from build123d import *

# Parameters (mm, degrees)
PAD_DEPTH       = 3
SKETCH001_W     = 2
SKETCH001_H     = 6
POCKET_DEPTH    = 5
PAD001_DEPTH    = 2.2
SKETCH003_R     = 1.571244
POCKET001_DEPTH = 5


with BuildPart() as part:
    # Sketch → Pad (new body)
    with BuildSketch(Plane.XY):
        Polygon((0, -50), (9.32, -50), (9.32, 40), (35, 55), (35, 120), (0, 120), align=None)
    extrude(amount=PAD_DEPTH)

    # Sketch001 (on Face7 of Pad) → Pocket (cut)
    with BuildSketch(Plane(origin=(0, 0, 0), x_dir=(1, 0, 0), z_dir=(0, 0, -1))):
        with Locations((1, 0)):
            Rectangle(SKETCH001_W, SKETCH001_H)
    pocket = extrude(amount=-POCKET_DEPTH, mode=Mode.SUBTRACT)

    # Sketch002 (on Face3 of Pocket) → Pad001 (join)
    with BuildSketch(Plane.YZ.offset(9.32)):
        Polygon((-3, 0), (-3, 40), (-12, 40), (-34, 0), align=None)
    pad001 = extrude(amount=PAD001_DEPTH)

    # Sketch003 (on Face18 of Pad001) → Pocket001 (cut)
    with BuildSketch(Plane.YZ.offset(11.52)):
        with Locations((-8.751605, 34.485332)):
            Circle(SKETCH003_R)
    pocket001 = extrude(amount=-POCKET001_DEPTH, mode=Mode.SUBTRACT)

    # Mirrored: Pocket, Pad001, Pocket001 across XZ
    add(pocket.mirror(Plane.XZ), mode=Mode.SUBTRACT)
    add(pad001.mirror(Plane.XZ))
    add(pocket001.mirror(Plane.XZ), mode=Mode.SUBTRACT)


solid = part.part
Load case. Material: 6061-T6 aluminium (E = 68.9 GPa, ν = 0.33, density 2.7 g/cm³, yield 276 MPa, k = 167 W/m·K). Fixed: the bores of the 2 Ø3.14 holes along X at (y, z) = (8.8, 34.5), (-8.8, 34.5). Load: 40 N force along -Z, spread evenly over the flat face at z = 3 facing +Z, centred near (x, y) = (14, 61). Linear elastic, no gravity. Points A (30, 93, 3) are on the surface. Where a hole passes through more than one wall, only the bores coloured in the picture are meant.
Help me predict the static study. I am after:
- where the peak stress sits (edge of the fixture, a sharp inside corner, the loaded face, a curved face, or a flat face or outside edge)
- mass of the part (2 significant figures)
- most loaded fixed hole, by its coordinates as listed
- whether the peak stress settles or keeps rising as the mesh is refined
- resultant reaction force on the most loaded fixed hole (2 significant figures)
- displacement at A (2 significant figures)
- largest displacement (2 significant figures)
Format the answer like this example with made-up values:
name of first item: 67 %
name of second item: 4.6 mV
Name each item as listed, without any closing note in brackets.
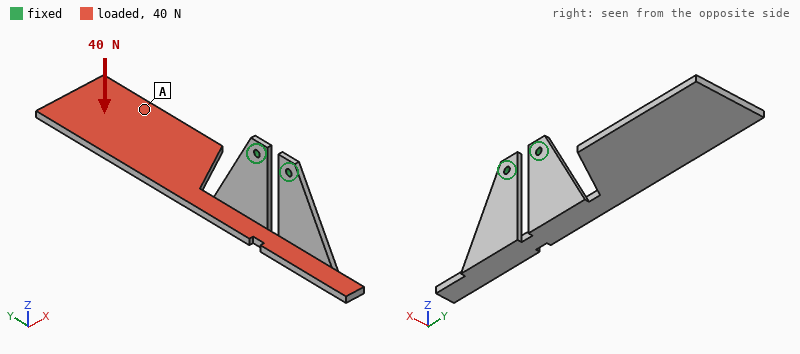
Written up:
where the peak stress sits: a sharp inside corner
mass of the part: 37 g
most loaded fixed hole, by its coordinates as listed: (8.8, 34.5)
whether the peak stress settles or keeps rising as the mesh is refined: keeps rising
resultant reaction force on the most loaded fixed hole: 83 N
displacement at A: 1.4 mm
largest displacement: 2.1 mm
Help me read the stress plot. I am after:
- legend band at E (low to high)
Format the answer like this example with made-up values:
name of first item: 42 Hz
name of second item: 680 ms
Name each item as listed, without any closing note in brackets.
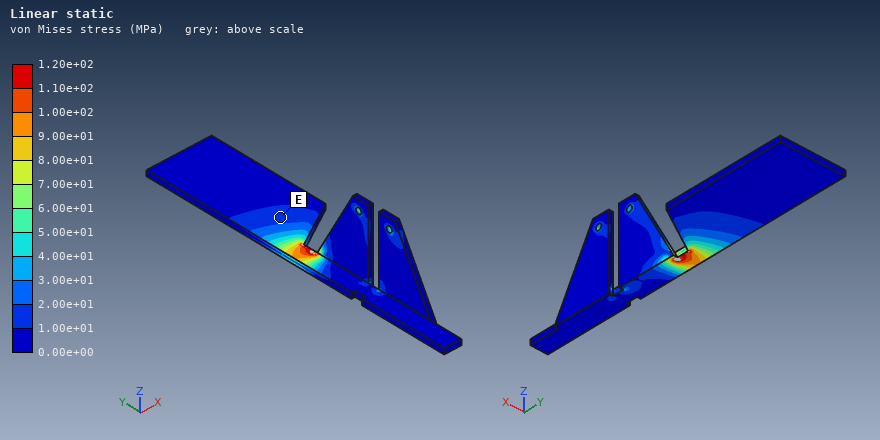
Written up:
legend band at E: 1.00e+01 to 2.00e+01 MPa
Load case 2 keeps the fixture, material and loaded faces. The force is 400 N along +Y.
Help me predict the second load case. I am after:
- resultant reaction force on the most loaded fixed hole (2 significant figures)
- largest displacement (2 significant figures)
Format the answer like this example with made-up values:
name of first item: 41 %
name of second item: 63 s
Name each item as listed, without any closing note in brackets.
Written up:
resultant reaction force on the most loaded fixed hole: 280 N
largest displacement: 1.9 mm
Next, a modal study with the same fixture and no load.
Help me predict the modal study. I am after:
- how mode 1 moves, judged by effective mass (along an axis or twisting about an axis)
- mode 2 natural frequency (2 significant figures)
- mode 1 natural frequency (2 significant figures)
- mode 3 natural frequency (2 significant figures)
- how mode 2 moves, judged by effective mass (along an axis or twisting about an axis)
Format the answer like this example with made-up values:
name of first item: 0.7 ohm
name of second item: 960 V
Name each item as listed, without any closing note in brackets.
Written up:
how mode 1 moves, judged by effective mass: along X
mode 2 natural frequency: 160 Hz
mode 1 natural frequency: 140 Hz
mode 3 natural frequency: 490 Hz
how mode 2 moves, judged by effective mass: along Z
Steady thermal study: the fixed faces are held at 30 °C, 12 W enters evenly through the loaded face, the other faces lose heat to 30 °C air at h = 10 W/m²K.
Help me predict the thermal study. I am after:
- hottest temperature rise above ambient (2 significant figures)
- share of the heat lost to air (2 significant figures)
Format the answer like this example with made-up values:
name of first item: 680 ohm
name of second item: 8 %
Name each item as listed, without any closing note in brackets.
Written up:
hottest temperature rise above ambient: 79 K
share of the heat lost to air: 26 %
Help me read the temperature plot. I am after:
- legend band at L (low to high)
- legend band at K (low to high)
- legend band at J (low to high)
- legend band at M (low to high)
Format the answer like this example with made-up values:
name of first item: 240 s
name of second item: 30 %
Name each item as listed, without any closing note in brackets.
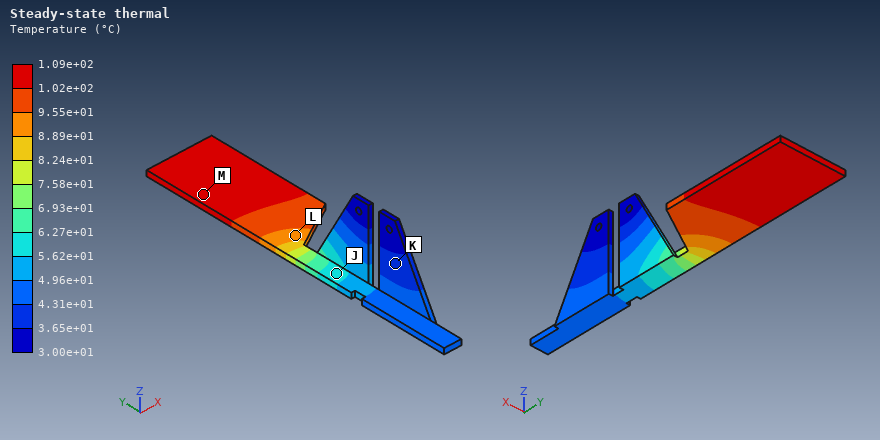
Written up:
legend band at L: 8.89e+01 to 9.55e+01 °C
legend band at K: 3.65e+01 to 4.31e+01 °C
legend band at J: 5.62e+01 to 6.27e+01 °C
legend band at M: 1.02e+02 to 1.09e+02 °C
